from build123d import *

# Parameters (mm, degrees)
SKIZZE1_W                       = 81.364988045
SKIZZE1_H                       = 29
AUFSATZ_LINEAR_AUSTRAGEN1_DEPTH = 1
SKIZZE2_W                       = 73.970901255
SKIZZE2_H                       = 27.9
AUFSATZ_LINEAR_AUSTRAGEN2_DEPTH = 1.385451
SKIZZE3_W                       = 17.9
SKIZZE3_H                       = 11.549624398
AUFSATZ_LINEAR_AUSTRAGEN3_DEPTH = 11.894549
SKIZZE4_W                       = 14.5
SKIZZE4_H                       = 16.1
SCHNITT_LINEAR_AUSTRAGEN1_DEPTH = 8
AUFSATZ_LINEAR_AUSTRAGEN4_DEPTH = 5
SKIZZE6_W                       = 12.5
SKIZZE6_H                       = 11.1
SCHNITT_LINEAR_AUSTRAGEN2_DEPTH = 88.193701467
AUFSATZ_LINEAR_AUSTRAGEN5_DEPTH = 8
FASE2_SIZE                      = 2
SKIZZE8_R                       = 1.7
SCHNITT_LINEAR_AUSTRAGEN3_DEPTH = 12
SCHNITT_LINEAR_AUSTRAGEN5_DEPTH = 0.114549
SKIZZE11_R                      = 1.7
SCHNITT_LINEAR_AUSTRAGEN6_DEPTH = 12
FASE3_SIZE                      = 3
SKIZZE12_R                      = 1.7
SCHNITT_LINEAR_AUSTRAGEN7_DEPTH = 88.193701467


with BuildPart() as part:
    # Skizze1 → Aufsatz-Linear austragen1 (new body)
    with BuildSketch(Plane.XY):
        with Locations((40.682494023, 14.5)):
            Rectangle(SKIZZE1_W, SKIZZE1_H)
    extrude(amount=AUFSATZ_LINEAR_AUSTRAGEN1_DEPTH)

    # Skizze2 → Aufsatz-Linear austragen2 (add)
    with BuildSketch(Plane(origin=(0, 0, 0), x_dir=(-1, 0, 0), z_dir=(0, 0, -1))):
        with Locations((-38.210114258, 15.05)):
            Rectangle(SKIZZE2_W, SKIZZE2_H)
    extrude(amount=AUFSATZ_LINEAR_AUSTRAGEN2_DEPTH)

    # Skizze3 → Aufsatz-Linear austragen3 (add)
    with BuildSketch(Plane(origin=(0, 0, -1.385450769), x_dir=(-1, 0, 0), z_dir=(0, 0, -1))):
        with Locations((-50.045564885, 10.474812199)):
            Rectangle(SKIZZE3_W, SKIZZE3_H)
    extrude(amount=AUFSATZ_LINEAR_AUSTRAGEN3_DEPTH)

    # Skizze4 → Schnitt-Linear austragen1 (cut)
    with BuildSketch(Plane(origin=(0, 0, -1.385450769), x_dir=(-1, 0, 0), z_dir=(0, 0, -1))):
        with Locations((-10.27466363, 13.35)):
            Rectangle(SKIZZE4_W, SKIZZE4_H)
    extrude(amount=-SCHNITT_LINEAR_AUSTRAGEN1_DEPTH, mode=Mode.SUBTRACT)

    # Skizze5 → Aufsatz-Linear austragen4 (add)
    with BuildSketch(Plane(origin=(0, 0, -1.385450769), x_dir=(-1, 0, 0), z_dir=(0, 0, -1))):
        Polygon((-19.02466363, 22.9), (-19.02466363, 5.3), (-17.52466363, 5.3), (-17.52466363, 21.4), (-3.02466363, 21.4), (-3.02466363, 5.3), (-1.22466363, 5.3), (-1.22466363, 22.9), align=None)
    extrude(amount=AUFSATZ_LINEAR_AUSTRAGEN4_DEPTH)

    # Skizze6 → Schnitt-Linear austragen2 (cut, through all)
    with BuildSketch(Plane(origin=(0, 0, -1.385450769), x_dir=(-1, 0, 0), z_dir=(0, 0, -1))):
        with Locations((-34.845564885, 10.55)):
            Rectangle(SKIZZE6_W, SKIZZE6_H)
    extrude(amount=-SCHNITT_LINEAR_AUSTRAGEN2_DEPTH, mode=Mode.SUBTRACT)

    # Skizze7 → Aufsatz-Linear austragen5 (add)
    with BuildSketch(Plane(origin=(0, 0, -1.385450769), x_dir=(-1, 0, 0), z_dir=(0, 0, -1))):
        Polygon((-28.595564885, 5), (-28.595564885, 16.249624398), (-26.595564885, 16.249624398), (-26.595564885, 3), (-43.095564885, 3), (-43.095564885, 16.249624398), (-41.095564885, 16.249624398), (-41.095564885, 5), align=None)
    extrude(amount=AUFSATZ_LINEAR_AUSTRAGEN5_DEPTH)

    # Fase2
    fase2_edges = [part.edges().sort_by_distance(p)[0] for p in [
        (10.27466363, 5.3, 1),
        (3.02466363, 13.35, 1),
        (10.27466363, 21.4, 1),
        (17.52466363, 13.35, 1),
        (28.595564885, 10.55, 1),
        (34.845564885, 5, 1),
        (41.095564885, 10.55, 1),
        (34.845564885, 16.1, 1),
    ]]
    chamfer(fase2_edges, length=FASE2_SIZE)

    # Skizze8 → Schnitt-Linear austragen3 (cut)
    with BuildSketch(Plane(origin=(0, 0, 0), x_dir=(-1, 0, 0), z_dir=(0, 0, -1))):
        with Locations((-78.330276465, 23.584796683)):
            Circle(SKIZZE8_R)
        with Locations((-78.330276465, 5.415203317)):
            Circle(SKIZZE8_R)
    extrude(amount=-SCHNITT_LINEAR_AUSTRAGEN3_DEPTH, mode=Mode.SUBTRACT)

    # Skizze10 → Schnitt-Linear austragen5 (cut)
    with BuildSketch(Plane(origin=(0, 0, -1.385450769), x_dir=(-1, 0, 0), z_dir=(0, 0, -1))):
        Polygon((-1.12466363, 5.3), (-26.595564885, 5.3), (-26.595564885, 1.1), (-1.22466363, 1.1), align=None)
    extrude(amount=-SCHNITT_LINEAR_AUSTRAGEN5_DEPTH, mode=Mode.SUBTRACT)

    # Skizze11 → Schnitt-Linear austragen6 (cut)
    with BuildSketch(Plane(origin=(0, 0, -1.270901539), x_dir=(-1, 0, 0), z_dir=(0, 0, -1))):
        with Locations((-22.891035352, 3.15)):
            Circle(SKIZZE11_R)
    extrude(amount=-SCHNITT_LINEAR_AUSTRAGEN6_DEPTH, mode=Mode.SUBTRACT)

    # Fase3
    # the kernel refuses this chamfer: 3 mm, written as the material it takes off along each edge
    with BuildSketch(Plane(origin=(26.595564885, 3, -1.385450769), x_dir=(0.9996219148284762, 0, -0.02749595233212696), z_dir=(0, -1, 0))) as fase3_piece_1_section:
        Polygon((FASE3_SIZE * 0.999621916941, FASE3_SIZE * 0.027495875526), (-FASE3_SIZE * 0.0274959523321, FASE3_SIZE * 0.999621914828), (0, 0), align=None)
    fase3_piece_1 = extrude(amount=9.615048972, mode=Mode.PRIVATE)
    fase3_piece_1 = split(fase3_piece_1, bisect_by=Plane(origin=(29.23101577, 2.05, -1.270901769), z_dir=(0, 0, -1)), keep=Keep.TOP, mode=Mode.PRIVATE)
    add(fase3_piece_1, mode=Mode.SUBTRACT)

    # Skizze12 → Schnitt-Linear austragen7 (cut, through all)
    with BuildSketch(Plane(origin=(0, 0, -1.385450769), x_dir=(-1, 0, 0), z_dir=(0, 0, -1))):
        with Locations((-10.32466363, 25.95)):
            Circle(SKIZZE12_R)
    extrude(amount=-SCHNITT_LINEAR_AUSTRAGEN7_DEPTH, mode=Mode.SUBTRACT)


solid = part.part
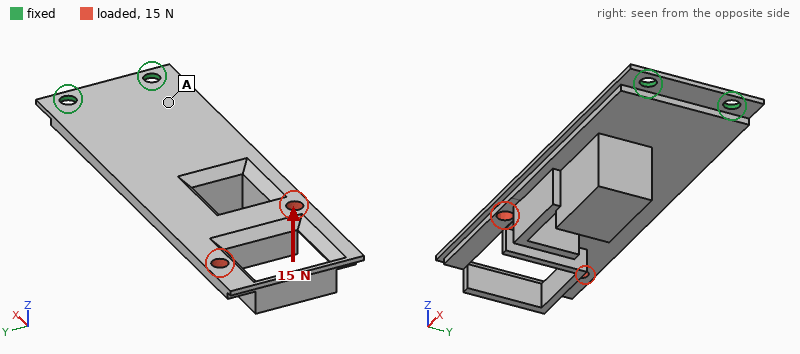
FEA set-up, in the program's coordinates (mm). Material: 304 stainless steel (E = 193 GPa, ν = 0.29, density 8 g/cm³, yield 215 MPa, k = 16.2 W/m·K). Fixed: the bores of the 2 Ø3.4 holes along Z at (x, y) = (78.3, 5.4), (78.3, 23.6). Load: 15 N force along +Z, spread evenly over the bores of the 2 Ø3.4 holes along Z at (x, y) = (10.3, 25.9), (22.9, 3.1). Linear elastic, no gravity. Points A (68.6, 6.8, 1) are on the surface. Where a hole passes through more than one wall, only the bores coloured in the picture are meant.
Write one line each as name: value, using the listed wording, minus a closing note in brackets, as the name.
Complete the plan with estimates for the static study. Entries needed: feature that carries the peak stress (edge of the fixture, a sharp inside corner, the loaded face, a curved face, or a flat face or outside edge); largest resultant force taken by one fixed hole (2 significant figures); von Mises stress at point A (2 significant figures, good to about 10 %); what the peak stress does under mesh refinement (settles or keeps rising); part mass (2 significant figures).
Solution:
feature that carries the peak stress: edge of the fixture
largest resultant force taken by one fixed hole: 12 N
von Mises stress at point A: 27 MPa
what the peak stress does under mesh refinement: keeps rising
part mass: 59 g
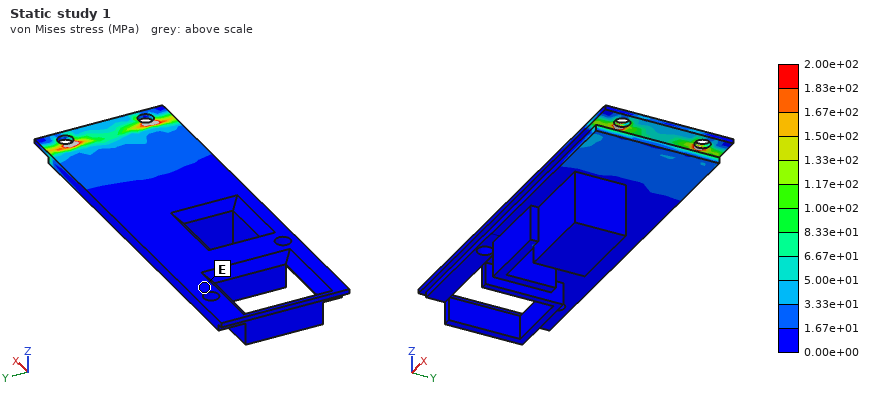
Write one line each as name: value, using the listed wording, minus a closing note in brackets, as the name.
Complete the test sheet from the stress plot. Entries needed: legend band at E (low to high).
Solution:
legend band at E: 0.00e+00 to 1.67e+01 MPa
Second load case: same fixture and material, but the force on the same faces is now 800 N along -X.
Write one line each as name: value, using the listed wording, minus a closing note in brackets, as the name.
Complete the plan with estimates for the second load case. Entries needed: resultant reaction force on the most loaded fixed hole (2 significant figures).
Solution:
resultant reaction force on the most loaded fixed hole: 420 N
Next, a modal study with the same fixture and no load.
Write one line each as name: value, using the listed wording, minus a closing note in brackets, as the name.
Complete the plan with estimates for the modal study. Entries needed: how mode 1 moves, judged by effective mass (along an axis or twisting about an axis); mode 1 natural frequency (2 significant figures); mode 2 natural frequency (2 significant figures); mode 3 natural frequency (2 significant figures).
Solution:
how mode 1 moves, judged by effective mass: along Z
mode 1 natural frequency: 200 Hz
mode 2 natural frequency: 1500 Hz
mode 3 natural frequency: 2000 Hz
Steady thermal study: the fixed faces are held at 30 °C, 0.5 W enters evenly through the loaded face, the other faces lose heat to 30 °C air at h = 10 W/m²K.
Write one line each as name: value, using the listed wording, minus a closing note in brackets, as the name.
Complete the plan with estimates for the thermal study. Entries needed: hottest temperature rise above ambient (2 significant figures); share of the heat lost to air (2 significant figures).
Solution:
hottest temperature rise above ambient: 16 K
share of the heat lost to air: 76 %
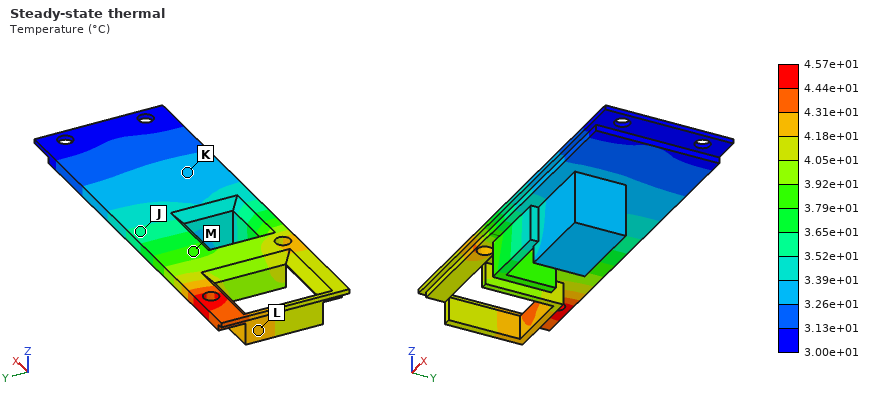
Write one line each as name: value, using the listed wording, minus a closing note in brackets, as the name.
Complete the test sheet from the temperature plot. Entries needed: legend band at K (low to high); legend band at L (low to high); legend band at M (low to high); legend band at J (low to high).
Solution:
legend band at K: 3.26e+01 to 3.39e+01 °C
legend band at L: 4.18e+01 to 4.31e+01 °C
legend band at M: 3.79e+01 to 3.92e+01 °C
legend band at J: 3.52e+01 to 3.65e+01 °C
